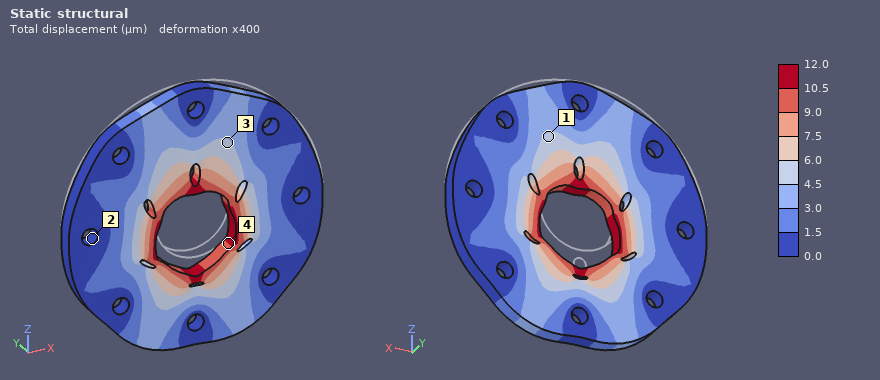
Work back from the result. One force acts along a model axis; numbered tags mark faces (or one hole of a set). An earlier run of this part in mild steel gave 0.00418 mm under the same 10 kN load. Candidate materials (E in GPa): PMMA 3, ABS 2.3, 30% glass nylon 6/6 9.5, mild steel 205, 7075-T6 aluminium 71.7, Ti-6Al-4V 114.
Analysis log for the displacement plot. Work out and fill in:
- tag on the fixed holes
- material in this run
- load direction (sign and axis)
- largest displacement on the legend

2
7075-T6 aluminium
-Z
12.0 µm
